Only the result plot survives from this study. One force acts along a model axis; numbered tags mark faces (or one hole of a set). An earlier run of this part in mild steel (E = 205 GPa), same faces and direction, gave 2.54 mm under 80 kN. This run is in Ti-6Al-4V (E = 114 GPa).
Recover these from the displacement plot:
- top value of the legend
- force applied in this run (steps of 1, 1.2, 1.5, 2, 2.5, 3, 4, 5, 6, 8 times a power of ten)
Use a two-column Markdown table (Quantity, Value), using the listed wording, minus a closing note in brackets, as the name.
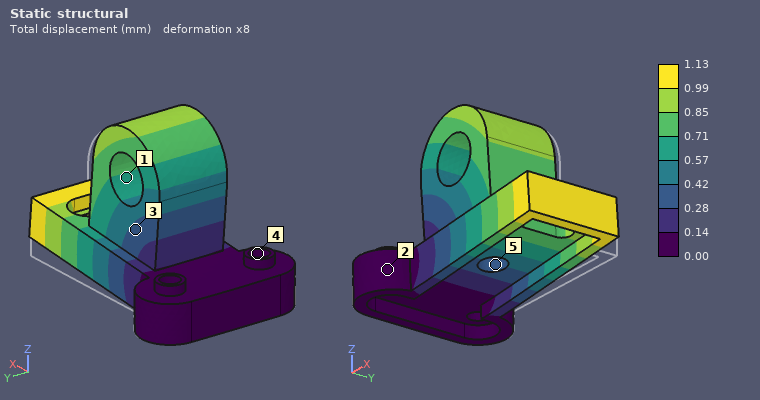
| Quantity | Value |
|---|---|
| top value of the legend | 1.13 mm |
| force applied in this run | 20 kN |
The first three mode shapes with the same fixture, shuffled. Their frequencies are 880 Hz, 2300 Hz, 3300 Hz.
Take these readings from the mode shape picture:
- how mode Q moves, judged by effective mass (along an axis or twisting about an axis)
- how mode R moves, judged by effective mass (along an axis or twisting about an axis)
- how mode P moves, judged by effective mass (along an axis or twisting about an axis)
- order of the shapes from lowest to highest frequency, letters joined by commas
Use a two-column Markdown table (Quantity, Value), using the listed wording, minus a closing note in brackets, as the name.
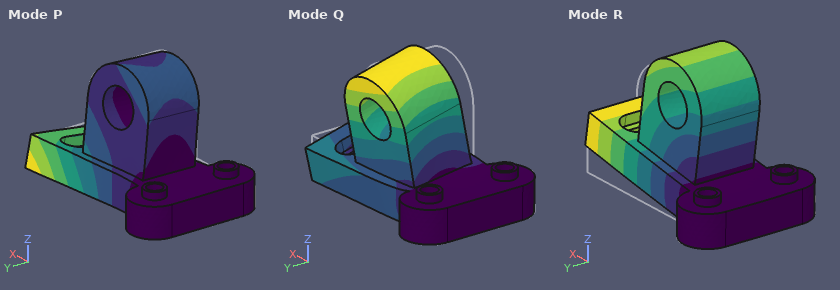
| Quantity | Value |
|---|---|
| how mode Q moves, judged by effective mass | along Y |
| how mode R moves, judged by effective mass | along Z |
| how mode P moves, judged by effective mass | along Y |
| order of the shapes from lowest to highest frequency, letters joined by commas | R, Q, P |
